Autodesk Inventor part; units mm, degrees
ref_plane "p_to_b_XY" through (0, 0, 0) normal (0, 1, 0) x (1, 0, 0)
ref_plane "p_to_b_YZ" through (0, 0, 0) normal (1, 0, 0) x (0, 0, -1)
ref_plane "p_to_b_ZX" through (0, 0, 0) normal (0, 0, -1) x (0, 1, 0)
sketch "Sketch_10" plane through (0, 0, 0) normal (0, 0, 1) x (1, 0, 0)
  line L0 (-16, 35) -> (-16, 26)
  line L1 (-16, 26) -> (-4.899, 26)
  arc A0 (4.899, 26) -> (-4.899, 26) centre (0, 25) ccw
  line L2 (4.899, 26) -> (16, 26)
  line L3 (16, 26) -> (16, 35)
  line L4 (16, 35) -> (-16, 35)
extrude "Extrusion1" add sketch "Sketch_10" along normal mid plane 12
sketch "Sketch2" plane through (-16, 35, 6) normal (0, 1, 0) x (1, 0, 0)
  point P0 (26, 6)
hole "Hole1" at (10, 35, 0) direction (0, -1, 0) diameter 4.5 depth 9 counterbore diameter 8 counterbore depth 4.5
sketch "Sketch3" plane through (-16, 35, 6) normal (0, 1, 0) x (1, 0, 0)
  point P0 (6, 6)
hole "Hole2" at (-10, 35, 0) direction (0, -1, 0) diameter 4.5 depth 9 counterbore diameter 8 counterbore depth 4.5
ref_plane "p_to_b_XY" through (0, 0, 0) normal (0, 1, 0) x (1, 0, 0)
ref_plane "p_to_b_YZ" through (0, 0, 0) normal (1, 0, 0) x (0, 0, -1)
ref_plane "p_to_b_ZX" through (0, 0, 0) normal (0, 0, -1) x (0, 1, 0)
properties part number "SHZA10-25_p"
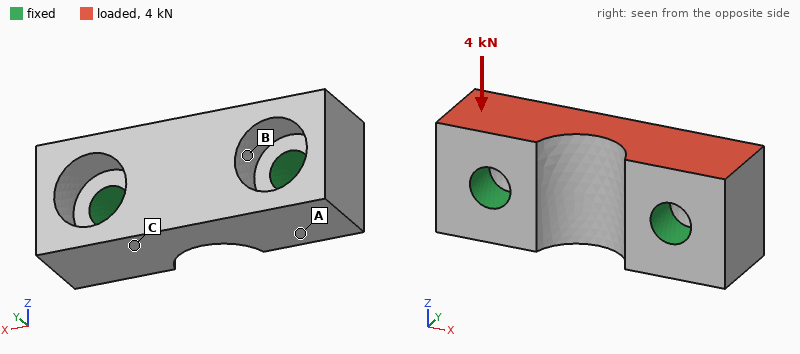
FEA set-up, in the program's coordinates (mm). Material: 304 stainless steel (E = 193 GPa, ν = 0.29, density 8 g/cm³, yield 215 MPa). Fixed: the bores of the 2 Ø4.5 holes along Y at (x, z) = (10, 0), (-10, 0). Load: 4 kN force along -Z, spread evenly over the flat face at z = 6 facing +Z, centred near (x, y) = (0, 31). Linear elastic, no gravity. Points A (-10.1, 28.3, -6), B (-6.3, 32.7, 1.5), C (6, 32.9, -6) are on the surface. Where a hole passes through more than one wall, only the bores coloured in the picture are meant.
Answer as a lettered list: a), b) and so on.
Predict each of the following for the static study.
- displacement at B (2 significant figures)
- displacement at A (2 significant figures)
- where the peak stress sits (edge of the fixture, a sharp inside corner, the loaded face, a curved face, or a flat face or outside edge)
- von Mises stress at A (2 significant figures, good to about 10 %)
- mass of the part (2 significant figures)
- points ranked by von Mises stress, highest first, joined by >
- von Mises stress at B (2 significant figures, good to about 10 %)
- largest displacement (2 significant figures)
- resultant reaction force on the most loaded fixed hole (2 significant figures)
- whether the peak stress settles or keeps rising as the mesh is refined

a) 3.2 µm
b) 1.3 µm
c) edge of the fixture
d) 24 MPa
e) 20 g
f) B > A > C
g) 46 MPa
h) 5.8 µm
i) 2.0 kN
j) keeps rising
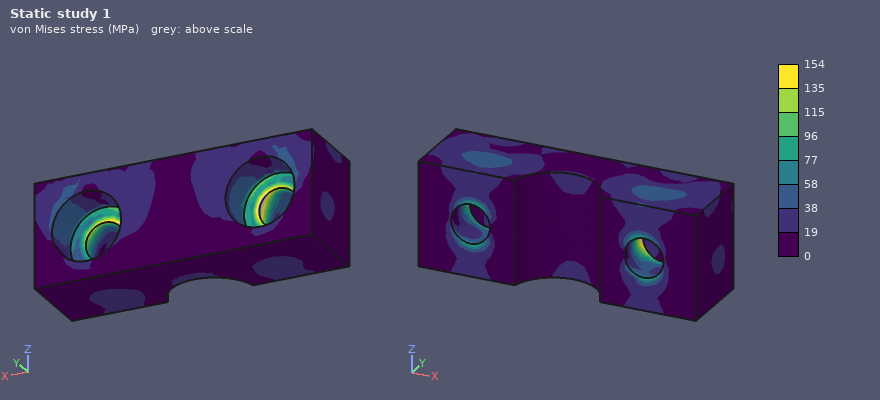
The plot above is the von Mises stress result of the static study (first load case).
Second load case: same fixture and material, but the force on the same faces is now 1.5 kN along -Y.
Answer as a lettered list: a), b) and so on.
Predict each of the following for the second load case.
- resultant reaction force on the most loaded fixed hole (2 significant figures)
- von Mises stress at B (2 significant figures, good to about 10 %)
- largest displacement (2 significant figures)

a) 760 N
b) 15 MPa
c) 3.8 µm
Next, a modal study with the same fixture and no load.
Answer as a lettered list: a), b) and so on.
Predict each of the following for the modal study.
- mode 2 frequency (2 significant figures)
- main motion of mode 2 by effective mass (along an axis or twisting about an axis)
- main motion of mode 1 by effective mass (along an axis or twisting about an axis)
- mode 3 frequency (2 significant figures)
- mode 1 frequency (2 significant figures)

a) 51 kHz
b) twisting about Y
c) along Z
d) 53 kHz
e) 36 kHz
